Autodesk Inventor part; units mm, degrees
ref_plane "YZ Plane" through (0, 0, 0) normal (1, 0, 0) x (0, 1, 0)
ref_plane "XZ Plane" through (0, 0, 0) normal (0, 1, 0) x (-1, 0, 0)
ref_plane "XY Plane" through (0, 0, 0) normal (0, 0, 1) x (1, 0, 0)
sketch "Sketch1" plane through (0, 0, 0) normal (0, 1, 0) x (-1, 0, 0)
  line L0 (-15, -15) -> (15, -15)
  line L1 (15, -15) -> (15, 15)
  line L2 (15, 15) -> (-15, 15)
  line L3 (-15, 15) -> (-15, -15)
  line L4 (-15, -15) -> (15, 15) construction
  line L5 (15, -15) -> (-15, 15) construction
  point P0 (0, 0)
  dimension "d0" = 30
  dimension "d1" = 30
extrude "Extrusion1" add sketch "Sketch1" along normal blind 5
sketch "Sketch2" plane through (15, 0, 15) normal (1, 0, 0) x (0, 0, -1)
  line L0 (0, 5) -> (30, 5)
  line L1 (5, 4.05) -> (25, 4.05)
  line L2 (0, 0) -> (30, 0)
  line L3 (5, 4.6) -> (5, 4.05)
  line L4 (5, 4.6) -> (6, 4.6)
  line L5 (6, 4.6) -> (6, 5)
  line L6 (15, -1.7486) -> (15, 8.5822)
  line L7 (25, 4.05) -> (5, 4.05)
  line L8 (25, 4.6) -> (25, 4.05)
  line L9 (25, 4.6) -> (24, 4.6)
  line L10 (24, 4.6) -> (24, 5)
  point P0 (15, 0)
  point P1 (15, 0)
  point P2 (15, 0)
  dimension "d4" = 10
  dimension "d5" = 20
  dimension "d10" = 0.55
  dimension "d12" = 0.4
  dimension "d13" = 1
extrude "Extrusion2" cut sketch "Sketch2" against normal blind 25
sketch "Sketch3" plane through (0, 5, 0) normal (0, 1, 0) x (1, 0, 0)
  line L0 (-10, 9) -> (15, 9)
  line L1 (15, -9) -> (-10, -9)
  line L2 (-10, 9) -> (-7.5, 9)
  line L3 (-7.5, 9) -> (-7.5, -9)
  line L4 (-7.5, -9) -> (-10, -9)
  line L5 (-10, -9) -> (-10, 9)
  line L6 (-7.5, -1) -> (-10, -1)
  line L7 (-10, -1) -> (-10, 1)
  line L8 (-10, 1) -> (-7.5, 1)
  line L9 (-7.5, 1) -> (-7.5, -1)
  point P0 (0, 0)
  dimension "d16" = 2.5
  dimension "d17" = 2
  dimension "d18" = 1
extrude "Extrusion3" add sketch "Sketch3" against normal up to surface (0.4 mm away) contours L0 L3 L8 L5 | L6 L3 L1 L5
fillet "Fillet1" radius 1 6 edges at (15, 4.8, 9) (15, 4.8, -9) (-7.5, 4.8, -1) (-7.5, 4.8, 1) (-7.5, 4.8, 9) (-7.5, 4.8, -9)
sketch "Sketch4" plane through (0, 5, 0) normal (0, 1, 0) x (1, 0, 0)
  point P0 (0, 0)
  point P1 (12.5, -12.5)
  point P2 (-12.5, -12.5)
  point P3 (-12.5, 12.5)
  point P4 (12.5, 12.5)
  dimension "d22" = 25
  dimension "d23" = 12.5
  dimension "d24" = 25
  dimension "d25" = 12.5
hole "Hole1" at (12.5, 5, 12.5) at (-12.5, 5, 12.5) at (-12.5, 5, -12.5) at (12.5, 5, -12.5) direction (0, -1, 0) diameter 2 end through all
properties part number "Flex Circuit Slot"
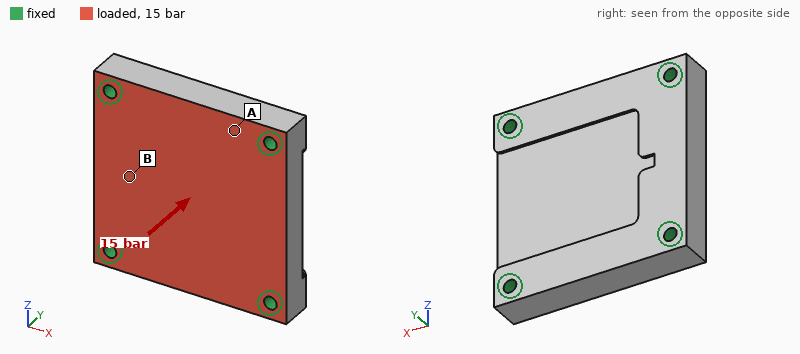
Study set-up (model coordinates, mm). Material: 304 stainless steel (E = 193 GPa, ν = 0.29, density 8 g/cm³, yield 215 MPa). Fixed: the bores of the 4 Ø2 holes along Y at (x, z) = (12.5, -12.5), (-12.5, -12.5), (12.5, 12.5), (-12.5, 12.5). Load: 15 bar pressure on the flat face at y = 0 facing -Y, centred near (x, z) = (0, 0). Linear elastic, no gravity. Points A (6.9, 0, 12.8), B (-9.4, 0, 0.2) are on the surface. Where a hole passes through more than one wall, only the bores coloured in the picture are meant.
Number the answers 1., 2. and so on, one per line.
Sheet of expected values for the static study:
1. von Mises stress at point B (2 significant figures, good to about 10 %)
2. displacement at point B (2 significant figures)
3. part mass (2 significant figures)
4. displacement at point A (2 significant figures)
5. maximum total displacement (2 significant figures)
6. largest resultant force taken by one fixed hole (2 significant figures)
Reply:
1. 14 MPa
2. 2.5 µm
3. 32 g
4. 1.2 µm
5. 3.7 µm
6. 340 N
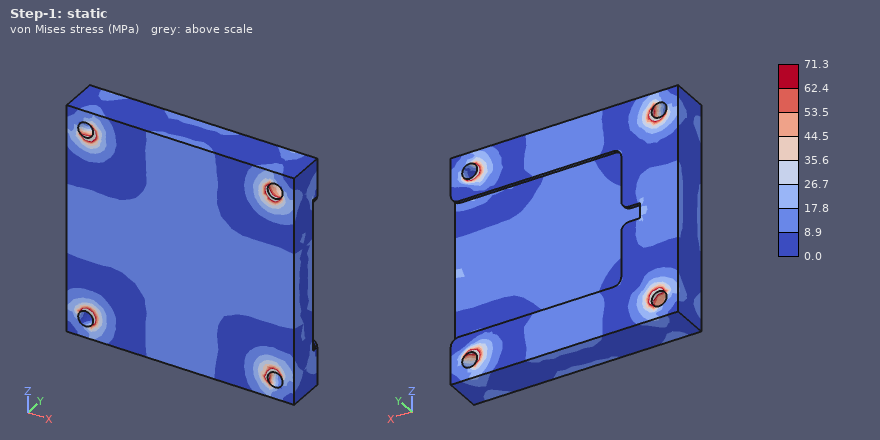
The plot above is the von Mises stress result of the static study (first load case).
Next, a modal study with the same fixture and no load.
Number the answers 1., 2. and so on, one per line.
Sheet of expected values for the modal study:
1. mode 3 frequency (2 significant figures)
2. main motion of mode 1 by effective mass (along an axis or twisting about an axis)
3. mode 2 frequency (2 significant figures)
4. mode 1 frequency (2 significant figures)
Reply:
1. 34 kHz
2. along Y
3. 33 kHz
4. 21 kHz
